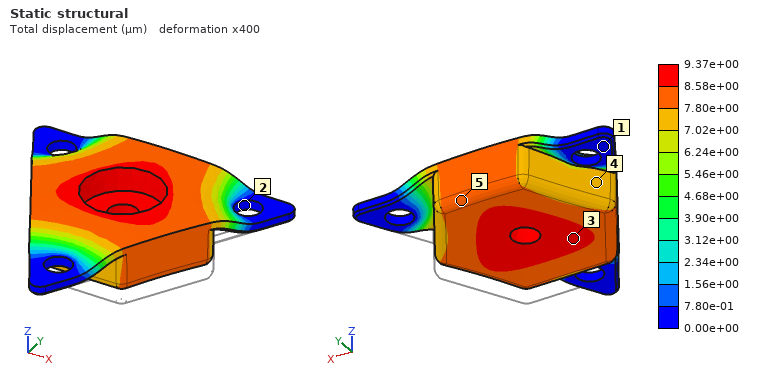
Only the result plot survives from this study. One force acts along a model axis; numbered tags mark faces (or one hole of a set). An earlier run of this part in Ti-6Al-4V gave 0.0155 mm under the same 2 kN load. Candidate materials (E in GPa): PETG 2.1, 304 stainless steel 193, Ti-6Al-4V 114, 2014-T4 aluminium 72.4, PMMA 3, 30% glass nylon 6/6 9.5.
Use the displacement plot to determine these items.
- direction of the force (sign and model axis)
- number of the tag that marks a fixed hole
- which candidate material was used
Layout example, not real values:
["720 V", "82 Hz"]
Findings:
["+Z", "2", "304 stainless steel"]
